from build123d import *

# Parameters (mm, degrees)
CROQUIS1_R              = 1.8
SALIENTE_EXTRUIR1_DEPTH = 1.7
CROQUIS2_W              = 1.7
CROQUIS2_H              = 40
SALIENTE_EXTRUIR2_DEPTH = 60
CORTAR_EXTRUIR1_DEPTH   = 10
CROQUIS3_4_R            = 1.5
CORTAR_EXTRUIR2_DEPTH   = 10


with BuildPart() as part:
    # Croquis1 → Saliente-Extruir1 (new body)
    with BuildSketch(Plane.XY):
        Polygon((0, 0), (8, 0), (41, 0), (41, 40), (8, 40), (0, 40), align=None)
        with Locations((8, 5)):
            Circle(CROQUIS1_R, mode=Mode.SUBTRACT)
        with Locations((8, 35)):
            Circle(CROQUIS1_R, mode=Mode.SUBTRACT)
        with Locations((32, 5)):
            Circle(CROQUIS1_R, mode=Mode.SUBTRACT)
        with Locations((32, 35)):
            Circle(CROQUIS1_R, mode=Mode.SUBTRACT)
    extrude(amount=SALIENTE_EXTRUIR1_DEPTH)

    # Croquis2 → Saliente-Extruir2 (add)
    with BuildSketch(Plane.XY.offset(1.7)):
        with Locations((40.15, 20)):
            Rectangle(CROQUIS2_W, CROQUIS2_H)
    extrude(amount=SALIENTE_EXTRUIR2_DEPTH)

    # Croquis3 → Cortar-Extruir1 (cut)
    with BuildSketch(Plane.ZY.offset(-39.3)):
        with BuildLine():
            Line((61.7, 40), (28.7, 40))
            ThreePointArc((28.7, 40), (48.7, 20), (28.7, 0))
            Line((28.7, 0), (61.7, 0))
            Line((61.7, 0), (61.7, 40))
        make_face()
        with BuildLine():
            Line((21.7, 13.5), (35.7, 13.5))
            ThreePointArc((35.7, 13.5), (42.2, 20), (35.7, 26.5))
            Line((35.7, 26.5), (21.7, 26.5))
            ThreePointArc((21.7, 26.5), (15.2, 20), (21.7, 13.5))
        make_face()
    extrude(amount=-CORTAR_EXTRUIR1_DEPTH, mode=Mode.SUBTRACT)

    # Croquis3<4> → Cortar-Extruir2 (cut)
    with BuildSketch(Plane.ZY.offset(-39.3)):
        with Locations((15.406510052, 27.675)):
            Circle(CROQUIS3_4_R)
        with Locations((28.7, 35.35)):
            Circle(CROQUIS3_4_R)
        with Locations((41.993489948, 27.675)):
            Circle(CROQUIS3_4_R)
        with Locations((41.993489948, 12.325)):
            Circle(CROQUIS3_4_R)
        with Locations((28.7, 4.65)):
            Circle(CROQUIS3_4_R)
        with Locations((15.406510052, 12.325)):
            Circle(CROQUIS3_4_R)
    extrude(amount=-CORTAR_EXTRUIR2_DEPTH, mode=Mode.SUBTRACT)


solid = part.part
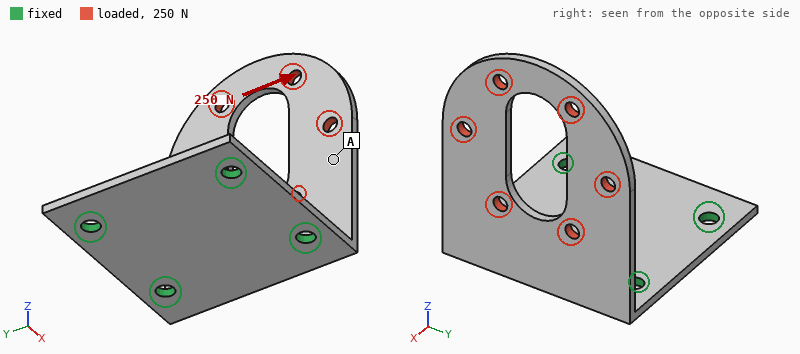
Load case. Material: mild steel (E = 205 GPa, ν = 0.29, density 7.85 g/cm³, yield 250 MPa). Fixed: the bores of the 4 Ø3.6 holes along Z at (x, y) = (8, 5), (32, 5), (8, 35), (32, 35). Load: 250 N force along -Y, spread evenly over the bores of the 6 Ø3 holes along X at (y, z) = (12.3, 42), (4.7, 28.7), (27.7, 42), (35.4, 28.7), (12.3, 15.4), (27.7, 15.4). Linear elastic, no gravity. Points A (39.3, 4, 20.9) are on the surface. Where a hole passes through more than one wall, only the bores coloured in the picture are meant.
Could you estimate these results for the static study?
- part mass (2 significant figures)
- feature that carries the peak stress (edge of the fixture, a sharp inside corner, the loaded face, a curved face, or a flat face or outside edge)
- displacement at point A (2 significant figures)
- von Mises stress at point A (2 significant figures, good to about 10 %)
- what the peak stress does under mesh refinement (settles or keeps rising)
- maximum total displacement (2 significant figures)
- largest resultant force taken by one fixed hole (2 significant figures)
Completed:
39 g
edge of the fixture
44 µm
18 MPa
keeps rising
68 µm
270 N
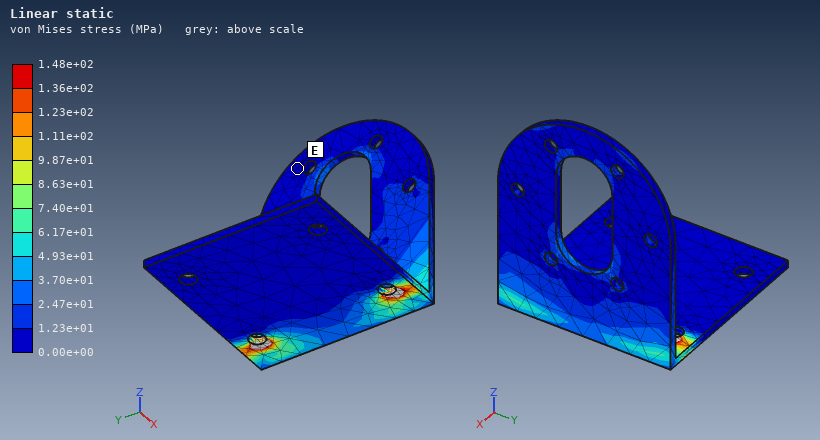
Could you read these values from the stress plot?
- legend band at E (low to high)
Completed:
0.00e+00 to 1.23e+01 MPa
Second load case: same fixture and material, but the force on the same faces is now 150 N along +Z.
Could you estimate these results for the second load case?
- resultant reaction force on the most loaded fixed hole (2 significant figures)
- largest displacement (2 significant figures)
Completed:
79 N
65 µm
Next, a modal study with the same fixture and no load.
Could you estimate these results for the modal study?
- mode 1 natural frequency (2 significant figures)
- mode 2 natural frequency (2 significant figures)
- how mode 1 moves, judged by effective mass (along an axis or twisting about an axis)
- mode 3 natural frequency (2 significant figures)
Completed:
630 Hz
1800 Hz
along X
3200 Hz
